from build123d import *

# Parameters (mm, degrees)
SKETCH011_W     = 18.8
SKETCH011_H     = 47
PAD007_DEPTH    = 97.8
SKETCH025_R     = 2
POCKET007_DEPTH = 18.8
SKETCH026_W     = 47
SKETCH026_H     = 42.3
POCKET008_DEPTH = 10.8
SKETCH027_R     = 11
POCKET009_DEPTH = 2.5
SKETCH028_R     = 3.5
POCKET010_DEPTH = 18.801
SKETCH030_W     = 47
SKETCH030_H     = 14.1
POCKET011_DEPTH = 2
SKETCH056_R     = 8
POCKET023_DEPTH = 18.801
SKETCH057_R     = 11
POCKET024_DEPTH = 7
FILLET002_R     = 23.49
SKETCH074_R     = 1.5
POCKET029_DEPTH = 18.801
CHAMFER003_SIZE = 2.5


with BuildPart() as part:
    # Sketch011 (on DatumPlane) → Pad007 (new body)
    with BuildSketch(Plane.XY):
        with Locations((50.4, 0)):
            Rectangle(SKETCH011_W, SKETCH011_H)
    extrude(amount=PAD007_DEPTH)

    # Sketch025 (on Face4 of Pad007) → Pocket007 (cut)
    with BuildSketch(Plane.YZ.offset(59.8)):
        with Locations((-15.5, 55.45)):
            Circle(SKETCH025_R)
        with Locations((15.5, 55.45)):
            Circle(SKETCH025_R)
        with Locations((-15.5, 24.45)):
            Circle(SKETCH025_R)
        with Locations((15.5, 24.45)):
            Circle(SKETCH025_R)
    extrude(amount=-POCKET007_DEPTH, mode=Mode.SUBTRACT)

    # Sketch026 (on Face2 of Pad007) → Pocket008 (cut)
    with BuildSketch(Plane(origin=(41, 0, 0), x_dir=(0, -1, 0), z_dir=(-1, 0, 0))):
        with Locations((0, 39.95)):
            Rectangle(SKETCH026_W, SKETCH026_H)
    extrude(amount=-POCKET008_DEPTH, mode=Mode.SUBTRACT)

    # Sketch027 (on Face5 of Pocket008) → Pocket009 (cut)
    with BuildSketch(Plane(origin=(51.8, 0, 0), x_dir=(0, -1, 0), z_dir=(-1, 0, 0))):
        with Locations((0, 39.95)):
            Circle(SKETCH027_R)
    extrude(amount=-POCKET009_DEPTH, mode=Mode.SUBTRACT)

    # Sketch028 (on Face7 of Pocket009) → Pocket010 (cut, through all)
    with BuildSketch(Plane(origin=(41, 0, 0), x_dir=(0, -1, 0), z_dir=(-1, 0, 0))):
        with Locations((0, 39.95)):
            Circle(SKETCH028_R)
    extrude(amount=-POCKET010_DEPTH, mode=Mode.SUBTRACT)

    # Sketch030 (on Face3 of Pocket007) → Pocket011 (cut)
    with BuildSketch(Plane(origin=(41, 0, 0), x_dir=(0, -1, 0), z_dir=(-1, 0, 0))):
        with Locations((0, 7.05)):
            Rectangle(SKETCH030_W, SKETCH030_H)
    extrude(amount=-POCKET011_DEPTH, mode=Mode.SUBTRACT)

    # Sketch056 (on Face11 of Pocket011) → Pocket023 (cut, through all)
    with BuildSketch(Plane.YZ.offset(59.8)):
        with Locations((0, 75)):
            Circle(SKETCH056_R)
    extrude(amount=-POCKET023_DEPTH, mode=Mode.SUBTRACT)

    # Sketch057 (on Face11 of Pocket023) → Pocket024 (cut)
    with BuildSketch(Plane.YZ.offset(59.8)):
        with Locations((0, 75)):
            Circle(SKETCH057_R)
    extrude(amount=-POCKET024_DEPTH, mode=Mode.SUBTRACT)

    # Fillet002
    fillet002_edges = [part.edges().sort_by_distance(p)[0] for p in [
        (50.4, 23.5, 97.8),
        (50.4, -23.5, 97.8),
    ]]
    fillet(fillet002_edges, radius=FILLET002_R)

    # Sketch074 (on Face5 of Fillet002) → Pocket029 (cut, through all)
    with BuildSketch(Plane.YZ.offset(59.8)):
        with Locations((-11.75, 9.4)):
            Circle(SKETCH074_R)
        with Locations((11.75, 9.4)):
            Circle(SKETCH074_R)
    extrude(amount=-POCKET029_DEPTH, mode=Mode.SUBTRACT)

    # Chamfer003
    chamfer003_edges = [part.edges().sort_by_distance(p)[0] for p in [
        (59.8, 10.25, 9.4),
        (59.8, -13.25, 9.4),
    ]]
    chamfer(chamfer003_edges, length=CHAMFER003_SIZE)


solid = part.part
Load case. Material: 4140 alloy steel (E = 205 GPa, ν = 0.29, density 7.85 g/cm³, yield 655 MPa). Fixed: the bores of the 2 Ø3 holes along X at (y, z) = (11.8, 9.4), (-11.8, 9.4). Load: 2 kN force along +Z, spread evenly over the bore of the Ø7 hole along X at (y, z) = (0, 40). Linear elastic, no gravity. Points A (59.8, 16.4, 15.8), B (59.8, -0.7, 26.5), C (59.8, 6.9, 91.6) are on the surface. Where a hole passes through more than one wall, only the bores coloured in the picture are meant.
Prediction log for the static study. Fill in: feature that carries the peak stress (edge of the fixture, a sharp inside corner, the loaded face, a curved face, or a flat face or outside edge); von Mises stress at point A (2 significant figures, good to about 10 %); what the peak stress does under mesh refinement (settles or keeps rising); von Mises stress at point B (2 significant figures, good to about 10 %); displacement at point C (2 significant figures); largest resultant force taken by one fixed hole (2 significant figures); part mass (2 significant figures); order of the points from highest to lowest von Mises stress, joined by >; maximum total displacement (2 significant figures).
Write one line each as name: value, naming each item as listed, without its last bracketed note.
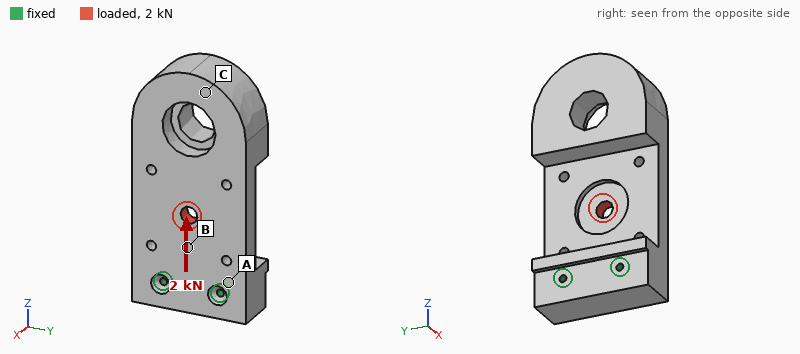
feature that carries the peak stress: edge of the fixture
von Mises stress at point A: 7.7 MPa
what the peak stress does under mesh refinement: keeps rising
von Mises stress at point B: 14 MPa
displacement at point C: 14 µm
largest resultant force taken by one fixed hole: 1.0 kN
part mass: 410 g
order of the points from highest to lowest von Mises stress, joined by >: B > A > C
maximum total displacement: 15 µm
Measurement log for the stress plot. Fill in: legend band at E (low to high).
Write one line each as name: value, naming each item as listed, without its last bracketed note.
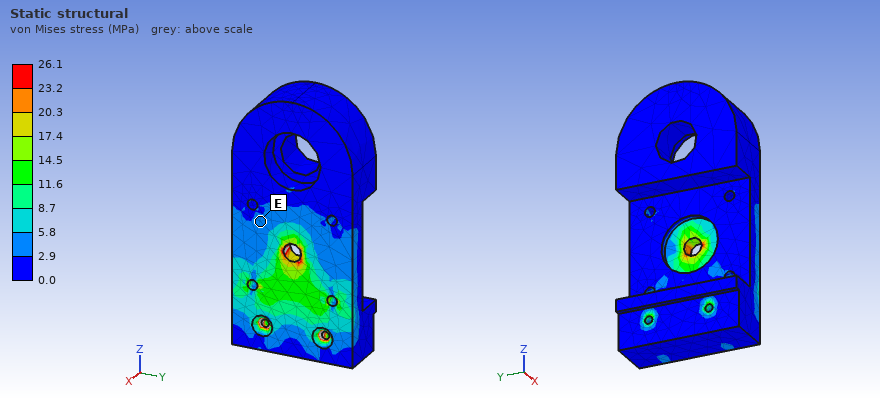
legend band at E: 2.9 to 5.8 MPa
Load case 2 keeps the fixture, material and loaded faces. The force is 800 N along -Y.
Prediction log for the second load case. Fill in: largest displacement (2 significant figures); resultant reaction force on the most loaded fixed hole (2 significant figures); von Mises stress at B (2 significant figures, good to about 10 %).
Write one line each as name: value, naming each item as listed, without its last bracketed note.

largest displacement: 4.7 µm
resultant reaction force on the most loaded fixed hole: 1.1 kN
von Mises stress at B: 6.4 MPa
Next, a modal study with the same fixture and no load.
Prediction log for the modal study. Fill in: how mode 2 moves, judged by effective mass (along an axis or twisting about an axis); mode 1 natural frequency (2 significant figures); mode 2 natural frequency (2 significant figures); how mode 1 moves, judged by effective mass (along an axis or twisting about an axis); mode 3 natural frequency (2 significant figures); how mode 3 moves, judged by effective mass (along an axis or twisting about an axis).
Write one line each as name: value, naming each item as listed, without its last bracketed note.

how mode 2 moves, judged by effective mass: along Y
mode 1 natural frequency: 690 Hz
mode 2 natural frequency: 2300 Hz
how mode 1 moves, judged by effective mass: along X
mode 3 natural frequency: 3400 Hz
how mode 3 moves, judged by effective mass: along Y
